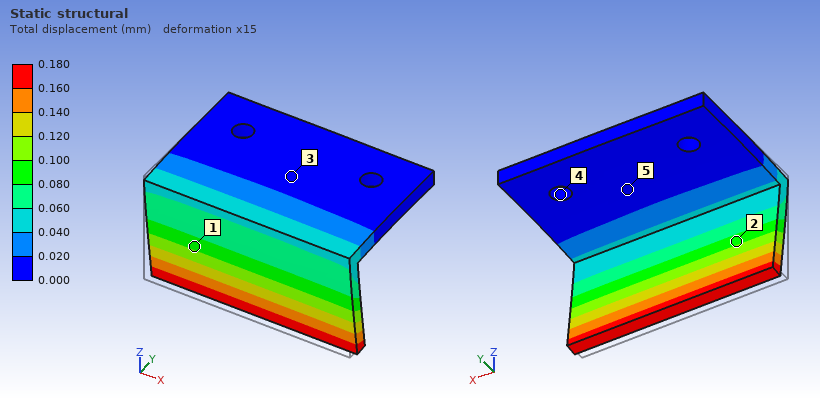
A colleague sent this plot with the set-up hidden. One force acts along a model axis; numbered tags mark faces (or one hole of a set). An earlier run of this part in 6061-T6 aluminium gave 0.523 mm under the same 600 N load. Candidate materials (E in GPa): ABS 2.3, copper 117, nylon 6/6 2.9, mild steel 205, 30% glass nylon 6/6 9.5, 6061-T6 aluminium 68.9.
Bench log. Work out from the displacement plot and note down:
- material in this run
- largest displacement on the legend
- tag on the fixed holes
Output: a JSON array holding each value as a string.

["mild steel", "0.180 mm", "4"]
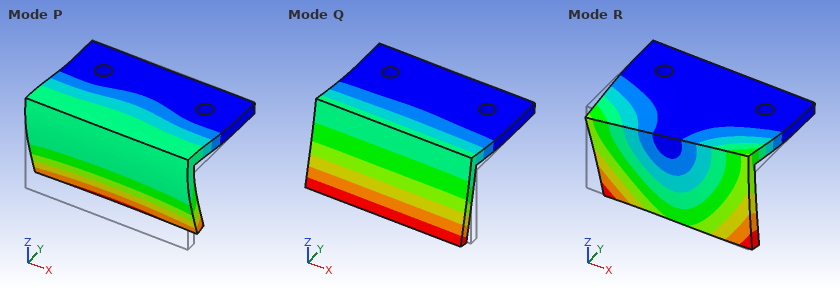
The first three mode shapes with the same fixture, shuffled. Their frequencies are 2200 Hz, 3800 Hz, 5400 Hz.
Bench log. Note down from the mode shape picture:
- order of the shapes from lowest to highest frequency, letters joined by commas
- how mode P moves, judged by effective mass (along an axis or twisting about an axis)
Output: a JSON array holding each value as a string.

["Q, R, P", "along Z"]
